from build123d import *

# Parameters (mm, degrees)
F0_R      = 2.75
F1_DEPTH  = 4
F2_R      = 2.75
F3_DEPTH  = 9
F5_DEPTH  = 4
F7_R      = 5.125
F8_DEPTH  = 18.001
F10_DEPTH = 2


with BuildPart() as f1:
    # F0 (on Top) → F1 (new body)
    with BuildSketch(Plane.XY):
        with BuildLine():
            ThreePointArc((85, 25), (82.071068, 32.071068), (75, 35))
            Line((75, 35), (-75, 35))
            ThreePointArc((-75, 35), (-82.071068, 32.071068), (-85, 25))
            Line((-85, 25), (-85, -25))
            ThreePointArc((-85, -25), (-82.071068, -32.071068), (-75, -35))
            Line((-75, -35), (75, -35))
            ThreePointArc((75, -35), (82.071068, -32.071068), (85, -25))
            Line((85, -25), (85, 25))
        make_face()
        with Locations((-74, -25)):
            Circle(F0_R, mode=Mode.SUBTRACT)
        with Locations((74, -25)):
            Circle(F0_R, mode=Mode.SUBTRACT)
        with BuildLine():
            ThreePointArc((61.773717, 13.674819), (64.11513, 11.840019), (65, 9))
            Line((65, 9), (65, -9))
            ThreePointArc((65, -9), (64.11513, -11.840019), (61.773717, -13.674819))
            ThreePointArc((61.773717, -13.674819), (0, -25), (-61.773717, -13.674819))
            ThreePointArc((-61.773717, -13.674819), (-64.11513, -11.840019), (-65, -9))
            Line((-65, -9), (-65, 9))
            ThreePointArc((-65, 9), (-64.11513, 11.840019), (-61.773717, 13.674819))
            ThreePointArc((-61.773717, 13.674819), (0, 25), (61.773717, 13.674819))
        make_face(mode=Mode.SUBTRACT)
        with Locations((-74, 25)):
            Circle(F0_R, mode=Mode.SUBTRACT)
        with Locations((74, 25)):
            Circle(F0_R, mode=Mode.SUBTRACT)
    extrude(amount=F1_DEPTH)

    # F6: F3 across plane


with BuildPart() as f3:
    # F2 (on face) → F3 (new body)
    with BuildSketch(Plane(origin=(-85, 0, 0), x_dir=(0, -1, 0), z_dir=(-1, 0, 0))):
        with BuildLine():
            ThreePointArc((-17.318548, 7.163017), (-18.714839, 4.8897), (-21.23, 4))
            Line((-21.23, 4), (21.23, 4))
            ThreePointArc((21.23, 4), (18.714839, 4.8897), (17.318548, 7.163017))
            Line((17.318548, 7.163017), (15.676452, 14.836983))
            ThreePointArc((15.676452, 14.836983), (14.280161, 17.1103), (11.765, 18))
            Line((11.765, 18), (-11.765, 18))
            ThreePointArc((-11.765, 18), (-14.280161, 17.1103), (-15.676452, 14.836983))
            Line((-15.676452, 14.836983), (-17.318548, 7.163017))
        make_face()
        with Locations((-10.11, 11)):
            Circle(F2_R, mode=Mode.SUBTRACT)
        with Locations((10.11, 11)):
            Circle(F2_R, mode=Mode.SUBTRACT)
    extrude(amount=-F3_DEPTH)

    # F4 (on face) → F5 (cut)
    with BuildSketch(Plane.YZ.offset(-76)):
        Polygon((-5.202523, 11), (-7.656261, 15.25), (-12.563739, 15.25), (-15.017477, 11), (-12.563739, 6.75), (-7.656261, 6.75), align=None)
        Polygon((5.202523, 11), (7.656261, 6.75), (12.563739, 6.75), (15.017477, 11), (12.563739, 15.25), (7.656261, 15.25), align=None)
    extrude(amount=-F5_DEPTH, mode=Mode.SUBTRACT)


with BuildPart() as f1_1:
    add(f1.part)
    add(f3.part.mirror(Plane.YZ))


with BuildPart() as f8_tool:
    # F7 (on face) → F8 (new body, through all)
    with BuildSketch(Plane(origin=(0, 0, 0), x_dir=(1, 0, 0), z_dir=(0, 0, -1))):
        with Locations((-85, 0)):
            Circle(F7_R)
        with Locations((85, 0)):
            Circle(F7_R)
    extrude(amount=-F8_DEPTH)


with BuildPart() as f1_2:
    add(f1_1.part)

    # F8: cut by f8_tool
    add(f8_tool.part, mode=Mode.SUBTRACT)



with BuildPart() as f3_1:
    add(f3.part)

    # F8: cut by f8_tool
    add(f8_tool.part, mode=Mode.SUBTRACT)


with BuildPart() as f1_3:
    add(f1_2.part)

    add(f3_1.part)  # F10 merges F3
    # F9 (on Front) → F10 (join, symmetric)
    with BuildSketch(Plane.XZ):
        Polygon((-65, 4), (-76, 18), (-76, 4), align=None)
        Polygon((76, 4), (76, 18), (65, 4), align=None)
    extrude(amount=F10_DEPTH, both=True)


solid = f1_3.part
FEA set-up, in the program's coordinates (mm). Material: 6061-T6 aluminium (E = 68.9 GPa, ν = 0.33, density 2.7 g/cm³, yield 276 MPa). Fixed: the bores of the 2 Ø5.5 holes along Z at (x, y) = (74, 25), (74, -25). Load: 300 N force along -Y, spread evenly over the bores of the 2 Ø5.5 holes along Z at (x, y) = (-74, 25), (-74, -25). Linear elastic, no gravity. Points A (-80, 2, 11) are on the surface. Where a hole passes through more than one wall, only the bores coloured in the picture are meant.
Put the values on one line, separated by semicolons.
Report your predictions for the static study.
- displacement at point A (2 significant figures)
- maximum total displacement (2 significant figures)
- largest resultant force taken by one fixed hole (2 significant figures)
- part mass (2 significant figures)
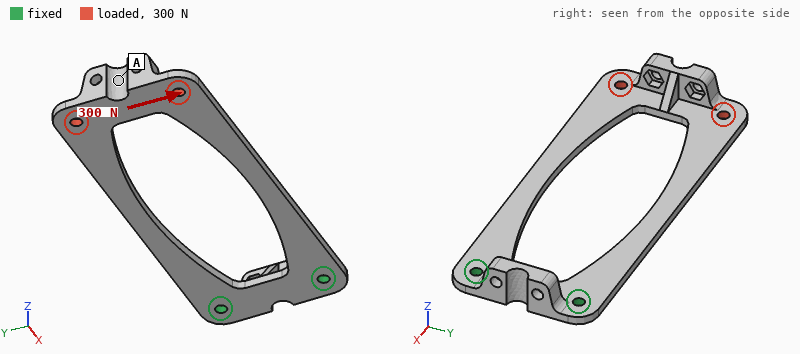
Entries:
0.43 mm; 0.44 mm; 770 N; 84 g
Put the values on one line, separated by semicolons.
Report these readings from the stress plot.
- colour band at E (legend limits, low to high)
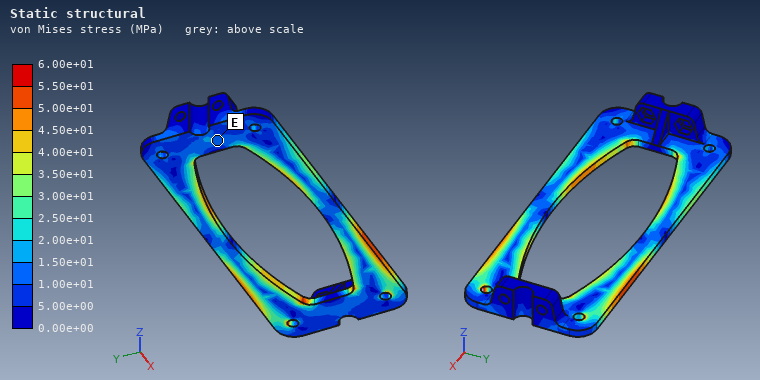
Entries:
1.00e+01 to 1.50e+01 MPa
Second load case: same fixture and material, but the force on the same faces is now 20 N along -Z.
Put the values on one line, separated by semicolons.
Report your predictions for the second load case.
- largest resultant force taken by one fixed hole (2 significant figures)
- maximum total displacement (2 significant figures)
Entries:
15 N; 2.2 mm
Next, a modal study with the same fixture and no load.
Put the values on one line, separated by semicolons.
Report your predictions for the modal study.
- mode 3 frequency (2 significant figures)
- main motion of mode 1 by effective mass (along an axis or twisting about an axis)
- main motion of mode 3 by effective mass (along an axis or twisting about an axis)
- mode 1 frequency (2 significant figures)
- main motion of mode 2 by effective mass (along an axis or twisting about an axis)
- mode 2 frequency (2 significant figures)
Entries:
690 Hz; along Z; along Y; 90 Hz; twisting about X; 410 Hz
